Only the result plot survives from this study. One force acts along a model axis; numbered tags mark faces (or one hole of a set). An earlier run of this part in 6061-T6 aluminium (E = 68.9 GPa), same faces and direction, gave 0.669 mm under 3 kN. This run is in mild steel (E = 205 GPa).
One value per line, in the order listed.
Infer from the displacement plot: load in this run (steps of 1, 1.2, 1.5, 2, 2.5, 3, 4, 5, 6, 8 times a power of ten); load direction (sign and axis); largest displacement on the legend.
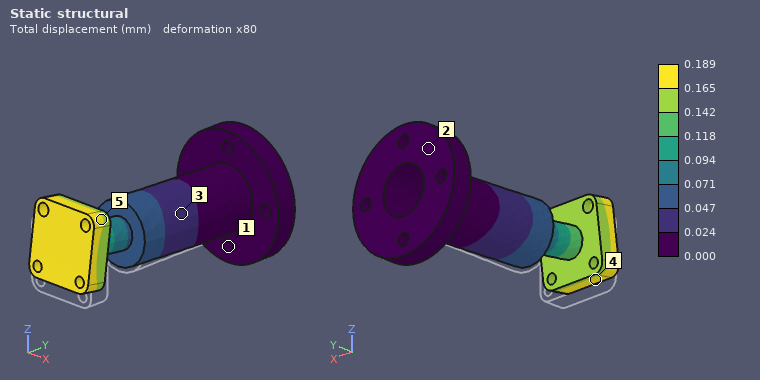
2.5 kN
+Z
0.189 mm
